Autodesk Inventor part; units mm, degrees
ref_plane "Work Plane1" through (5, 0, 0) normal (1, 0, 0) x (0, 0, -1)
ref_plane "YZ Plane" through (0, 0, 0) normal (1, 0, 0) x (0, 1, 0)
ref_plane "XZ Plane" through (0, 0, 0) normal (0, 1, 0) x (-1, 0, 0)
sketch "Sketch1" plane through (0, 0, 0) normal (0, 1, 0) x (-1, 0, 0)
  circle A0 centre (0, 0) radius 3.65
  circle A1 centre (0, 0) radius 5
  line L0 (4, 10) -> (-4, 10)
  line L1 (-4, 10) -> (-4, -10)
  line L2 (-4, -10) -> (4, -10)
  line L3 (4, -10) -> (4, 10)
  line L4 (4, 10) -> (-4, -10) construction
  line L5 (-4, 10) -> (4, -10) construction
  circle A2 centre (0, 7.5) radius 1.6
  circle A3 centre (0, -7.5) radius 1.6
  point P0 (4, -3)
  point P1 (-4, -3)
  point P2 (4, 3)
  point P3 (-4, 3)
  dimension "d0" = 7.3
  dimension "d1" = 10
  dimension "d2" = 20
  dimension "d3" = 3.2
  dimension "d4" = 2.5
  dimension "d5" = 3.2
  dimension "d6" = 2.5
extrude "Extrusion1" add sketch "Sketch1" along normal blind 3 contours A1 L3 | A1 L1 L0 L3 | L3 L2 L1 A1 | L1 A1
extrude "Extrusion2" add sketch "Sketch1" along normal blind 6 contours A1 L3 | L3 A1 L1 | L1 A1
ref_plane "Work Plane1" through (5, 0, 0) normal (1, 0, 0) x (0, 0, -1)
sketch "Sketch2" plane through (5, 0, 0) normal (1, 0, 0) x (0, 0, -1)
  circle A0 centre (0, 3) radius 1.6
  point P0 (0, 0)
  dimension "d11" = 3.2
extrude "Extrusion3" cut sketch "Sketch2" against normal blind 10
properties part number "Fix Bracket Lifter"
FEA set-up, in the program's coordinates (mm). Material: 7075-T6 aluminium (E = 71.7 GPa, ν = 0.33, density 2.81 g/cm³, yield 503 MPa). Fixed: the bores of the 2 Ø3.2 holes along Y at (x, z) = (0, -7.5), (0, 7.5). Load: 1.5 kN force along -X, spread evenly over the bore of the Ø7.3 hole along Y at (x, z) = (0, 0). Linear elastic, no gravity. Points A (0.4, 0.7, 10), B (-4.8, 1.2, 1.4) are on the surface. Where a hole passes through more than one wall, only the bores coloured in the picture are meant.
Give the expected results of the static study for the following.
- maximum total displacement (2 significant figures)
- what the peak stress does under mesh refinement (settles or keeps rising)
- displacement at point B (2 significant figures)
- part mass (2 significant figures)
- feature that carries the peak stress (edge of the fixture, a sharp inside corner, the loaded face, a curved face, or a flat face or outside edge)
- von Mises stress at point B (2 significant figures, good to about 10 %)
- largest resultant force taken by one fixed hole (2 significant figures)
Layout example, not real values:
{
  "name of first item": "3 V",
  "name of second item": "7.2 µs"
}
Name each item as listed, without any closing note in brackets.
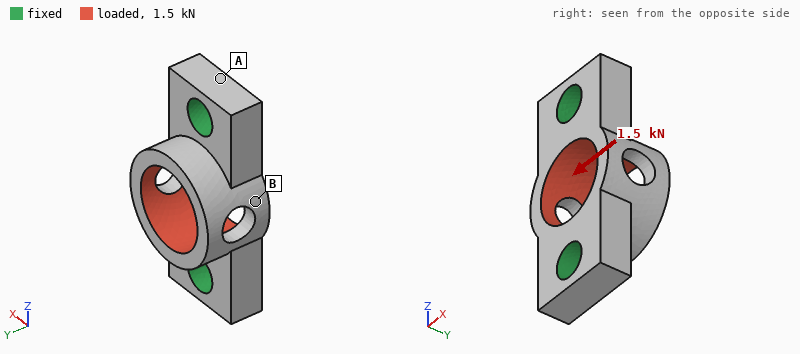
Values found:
{
  "maximum total displacement": "23 µm",
  "what the peak stress does under mesh refinement": "keeps rising",
  "displacement at point B": "12 µm",
  "part mass": "1.2 g",
  "feature that carries the peak stress": "edge of the fixture",
  "von Mises stress at point B": "67 MPa",
  "largest resultant force taken by one fixed hole": "750 N"
}
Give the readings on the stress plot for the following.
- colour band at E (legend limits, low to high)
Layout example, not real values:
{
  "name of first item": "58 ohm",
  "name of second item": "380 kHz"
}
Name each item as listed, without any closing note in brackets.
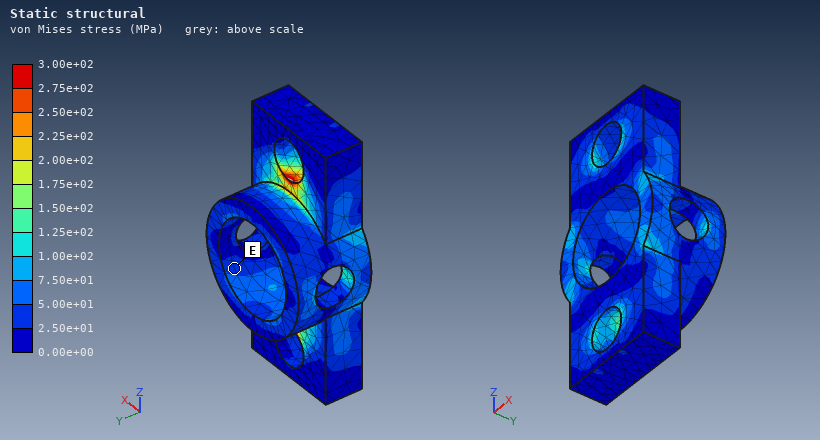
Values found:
{
  "colour band at E": "2.50e+01 to 5.00e+01 MPa"
}
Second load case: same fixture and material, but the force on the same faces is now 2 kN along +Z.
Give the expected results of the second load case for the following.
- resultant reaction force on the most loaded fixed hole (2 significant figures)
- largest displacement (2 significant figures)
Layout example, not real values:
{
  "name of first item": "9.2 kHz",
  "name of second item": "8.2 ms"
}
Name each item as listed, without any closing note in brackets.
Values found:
{
  "resultant reaction force on the most loaded fixed hole": "1.0 kN",
  "largest displacement": "13 µm"
}
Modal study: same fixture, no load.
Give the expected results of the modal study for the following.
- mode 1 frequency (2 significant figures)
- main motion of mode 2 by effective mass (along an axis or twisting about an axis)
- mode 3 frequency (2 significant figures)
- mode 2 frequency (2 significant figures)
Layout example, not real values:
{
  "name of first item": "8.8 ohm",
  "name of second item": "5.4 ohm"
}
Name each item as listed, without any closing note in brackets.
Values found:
{
  "mode 1 frequency": "53 kHz",
  "main motion of mode 2 by effective mass": "along Y",
  "mode 3 frequency": "79 kHz",
  "mode 2 frequency": "63 kHz"
}
